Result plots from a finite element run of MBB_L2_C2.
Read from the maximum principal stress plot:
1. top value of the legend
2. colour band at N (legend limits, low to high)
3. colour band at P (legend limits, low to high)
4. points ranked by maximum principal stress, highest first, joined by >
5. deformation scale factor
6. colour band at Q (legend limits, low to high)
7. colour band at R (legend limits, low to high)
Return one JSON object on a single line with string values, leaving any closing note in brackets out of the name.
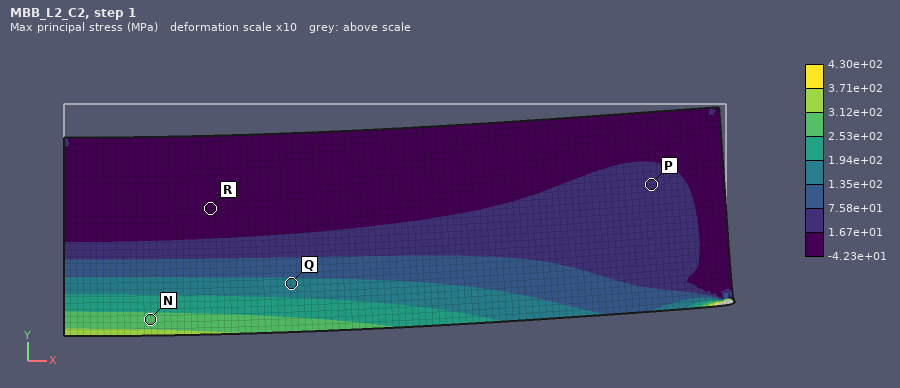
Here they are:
{"top value of the legend": "4.30e+02 MPa", "colour band at N": "2.53e+02 to 3.12e+02 MPa", "colour band at P": "1.67e+01 to 7.58e+01 MPa", "points ranked by maximum principal stress, highest first, joined by >": "N > Q > P > R", "deformation scale factor": "10", "colour band at Q": "1.35e+02 to 1.94e+02 MPa", "colour band at R": "-4.23e+01 to 1.67e+01 MPa"}
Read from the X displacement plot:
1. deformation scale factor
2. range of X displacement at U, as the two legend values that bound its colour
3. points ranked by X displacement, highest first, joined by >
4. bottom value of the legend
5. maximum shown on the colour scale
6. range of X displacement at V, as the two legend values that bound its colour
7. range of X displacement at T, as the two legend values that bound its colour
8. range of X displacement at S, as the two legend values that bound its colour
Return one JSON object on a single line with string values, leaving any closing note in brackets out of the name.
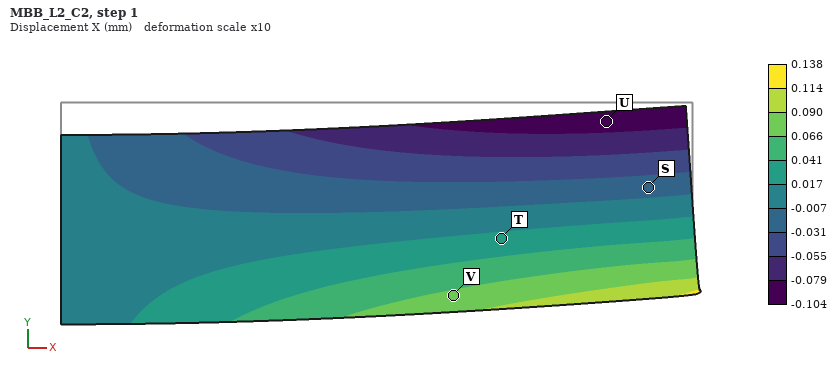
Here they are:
{"deformation scale factor": "10", "range of X displacement at U, as the two legend values that bound its colour": "-0.104 to -0.079 mm", "points ranked by X displacement, highest first, joined by >": "V > T > S > U", "bottom value of the legend": "-0.104 mm", "maximum shown on the colour scale": "0.138 mm", "range of X displacement at V, as the two legend values that bound its colour": "0.066 to 0.090 mm", "range of X displacement at T, as the two legend values that bound its colour": "0.017 to 0.041 mm", "range of X displacement at S, as the two legend values that bound its colour": "-0.031 to -0.007 mm"}
